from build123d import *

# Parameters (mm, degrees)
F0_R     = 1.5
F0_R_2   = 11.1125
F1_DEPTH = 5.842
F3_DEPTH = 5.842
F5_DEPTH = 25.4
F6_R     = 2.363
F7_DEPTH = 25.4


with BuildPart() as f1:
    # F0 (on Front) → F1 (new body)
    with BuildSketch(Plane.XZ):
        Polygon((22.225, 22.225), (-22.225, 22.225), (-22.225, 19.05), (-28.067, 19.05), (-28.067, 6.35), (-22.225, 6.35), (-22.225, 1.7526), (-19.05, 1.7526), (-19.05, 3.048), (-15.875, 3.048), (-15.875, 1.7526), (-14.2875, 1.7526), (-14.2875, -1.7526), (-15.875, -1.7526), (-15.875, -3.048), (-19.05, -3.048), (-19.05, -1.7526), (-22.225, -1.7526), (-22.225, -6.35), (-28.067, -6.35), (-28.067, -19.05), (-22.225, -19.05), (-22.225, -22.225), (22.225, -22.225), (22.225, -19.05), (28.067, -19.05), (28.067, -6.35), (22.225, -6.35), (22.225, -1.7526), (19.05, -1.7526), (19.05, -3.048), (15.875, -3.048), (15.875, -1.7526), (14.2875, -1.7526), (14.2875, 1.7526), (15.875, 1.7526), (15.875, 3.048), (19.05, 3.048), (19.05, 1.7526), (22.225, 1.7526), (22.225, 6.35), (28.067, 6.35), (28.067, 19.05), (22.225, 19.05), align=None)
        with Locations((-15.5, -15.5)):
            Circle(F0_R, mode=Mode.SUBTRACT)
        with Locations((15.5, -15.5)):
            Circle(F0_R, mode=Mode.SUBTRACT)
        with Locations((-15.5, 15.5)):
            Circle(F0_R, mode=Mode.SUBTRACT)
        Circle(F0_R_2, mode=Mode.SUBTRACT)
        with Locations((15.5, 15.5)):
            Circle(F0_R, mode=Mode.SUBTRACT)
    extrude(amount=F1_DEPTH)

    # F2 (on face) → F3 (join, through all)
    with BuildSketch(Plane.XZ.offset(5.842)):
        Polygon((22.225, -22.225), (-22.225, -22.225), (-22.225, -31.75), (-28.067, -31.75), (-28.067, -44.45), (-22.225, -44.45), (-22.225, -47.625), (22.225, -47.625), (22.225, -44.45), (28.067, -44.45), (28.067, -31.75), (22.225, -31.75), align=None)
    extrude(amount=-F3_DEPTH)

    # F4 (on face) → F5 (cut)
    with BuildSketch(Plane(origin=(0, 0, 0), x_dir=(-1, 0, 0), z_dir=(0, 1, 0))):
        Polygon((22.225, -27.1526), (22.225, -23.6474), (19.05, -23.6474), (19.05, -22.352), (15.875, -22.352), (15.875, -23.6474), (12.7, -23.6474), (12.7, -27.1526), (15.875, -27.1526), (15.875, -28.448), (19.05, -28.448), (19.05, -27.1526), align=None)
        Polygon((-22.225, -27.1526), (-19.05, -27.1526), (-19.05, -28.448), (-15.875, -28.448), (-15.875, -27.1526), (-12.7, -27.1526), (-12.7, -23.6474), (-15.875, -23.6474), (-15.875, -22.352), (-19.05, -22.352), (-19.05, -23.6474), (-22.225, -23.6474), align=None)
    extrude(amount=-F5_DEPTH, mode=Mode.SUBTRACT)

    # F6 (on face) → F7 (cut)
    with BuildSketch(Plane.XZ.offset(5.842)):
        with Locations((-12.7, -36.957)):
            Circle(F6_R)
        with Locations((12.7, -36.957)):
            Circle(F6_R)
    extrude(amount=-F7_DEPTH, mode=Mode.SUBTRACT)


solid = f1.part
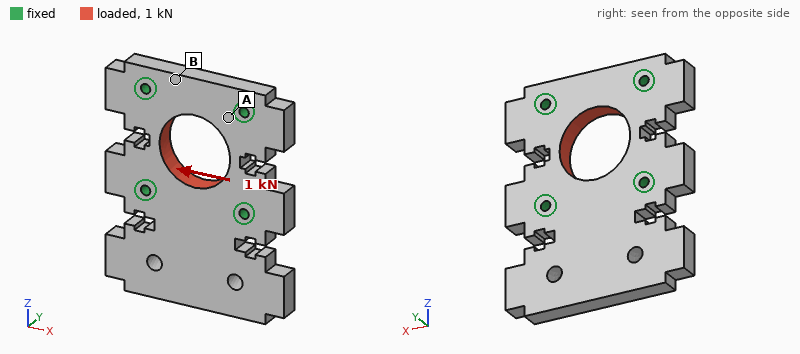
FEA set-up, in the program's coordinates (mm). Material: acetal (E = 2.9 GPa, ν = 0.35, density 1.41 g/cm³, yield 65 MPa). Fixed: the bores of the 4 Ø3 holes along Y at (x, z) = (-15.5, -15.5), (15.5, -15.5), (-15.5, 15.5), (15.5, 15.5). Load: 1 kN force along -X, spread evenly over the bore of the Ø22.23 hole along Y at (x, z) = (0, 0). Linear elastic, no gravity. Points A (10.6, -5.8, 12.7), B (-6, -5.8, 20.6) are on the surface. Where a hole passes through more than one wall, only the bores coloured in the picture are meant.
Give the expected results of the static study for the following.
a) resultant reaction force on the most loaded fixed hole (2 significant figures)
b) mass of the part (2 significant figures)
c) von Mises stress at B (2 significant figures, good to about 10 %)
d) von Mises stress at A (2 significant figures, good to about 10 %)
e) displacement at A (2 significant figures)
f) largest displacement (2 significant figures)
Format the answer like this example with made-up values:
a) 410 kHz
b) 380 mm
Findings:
a) 290 N
b) 24 g
c) 1.7 MPa
d) 3.8 MPa
e) 10 µm
f) 48 µm
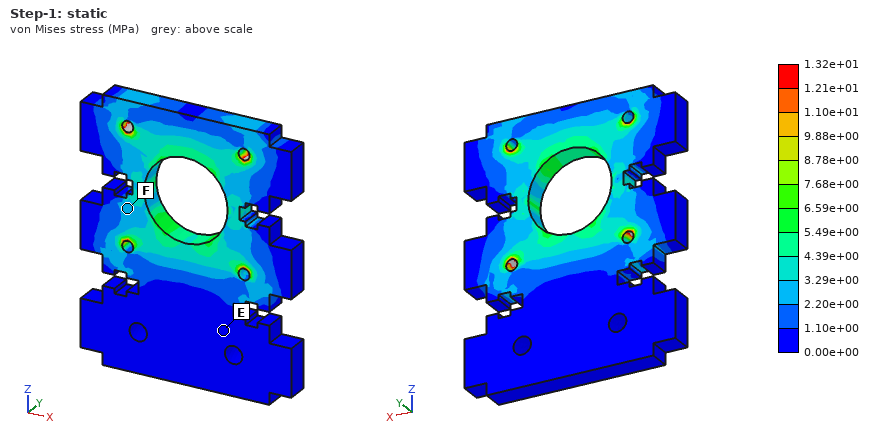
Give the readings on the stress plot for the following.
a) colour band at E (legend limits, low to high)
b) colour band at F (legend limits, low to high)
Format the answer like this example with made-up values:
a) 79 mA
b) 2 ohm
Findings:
a) 0.00e+00 to 1.10e+00 MPa
b) 2.20e+00 to 3.29e+00 MPa
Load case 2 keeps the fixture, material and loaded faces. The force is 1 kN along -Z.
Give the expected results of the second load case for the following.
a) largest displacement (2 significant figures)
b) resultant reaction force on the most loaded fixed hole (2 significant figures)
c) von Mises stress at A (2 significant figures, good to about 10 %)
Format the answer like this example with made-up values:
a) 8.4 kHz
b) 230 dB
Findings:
a) 45 µm
b) 270 N
c) 3.5 MPa
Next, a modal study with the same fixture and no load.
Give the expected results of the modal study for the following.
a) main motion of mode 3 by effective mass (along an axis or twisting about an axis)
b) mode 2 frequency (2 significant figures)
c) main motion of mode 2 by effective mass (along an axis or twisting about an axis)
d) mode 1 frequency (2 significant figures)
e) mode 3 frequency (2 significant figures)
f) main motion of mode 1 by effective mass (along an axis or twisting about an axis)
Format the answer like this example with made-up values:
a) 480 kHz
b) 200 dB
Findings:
a) along X
b) 1300 Hz
c) twisting about Z
d) 840 Hz
e) 2800 Hz
f) along Y
